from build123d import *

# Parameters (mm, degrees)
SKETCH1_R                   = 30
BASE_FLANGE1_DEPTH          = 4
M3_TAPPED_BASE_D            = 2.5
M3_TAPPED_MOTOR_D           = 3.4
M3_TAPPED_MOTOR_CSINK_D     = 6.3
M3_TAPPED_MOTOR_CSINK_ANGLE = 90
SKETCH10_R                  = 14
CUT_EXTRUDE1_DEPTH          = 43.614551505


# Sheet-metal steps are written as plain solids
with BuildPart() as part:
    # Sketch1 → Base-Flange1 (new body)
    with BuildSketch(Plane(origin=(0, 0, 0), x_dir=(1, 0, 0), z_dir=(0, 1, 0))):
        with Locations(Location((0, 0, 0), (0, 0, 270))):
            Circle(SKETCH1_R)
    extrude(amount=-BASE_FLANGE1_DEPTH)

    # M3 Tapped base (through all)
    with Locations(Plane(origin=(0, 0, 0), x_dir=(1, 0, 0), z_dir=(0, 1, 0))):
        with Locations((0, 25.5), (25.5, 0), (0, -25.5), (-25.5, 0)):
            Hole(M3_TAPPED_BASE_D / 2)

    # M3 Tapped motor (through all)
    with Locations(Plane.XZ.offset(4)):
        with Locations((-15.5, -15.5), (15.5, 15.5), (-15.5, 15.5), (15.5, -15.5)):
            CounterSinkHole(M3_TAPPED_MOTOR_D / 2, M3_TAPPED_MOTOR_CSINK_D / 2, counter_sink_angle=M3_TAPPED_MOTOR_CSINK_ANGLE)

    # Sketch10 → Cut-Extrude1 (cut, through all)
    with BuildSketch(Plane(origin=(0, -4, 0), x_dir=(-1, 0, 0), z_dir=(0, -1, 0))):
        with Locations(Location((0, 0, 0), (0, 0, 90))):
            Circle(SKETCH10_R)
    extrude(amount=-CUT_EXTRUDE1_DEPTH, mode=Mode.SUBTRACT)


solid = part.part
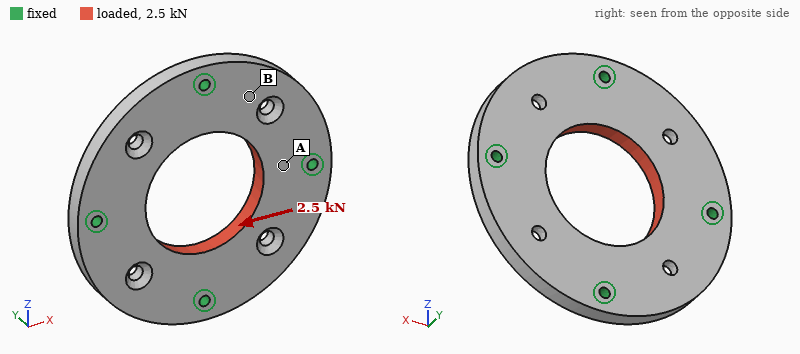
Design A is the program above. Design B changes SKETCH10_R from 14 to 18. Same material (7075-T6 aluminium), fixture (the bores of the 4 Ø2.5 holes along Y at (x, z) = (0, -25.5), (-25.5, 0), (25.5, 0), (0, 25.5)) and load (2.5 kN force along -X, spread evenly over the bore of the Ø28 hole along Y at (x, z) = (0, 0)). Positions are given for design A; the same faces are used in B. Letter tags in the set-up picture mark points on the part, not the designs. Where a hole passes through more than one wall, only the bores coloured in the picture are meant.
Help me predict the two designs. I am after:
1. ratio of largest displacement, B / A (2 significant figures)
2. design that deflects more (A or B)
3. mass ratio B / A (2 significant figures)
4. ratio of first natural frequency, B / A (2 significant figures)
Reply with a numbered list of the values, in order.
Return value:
1. 1.1
2. B
3. 0.81
4. 0.99
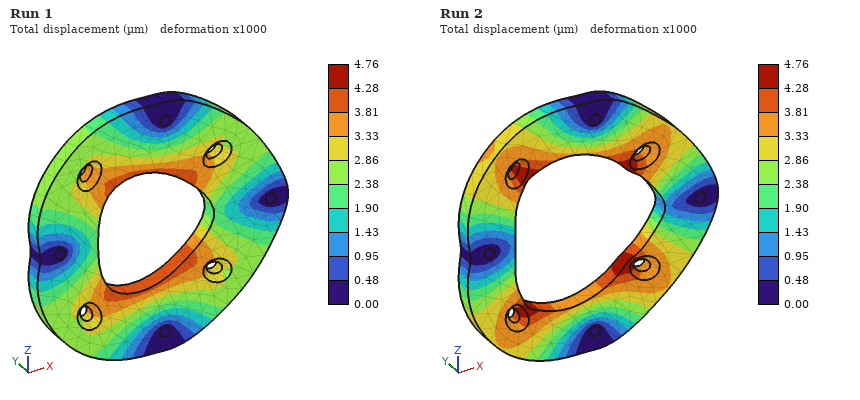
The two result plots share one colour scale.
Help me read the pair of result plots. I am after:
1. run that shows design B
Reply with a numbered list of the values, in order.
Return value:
1. Run 2
